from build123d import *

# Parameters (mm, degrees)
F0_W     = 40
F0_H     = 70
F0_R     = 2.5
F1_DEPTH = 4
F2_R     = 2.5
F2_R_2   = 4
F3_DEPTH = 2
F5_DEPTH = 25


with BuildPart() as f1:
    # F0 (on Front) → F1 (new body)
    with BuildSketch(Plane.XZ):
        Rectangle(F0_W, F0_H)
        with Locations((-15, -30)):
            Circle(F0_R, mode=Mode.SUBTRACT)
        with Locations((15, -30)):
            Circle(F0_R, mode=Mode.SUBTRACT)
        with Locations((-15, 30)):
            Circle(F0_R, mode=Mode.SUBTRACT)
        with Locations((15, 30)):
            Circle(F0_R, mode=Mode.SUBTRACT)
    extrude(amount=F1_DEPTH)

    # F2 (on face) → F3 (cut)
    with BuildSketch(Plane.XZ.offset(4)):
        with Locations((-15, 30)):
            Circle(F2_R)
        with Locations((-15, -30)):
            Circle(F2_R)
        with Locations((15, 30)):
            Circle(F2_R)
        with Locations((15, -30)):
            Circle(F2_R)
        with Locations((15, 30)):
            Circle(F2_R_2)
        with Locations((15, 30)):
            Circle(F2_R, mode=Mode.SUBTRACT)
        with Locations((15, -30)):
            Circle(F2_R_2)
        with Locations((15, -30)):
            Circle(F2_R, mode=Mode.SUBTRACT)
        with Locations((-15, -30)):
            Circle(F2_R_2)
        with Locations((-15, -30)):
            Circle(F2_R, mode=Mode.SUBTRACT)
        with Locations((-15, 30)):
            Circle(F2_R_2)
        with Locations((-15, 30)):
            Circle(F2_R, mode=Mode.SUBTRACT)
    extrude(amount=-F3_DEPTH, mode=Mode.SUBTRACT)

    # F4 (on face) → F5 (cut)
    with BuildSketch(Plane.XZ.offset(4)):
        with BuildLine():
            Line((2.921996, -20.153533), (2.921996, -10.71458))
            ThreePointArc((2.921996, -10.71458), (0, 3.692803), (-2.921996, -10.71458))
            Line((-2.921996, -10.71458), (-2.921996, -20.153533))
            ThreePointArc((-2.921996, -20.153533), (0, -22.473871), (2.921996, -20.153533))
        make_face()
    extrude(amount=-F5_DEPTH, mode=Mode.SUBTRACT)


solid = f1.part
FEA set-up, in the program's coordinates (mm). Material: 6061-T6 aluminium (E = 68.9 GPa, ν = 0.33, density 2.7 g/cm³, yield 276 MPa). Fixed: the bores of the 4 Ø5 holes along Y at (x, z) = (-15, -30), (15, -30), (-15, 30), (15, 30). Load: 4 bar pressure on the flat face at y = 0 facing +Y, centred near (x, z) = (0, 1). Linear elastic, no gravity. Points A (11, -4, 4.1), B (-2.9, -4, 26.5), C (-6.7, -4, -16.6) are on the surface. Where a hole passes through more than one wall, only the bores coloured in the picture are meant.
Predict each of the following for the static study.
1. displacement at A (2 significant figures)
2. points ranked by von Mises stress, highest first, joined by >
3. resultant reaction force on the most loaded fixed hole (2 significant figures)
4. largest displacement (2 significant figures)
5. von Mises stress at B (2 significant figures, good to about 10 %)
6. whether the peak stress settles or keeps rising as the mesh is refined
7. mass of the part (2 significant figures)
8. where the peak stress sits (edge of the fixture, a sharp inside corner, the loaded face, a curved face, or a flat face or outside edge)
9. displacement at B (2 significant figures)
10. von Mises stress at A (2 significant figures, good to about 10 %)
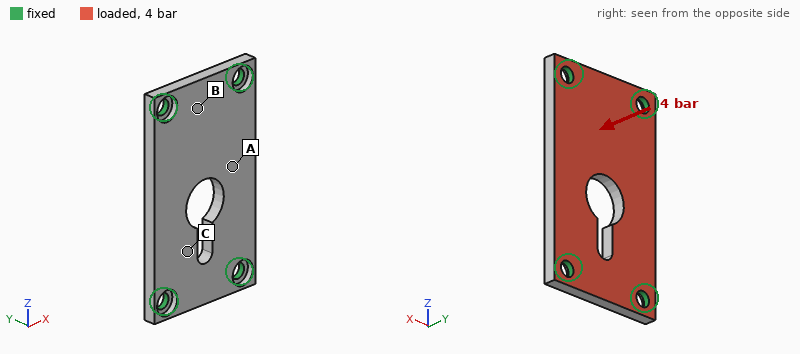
54 µm
A > B > C
360 N
60 µm
15 MPa
keeps rising
26 g
edge of the fixture
12 µm
29 MPa
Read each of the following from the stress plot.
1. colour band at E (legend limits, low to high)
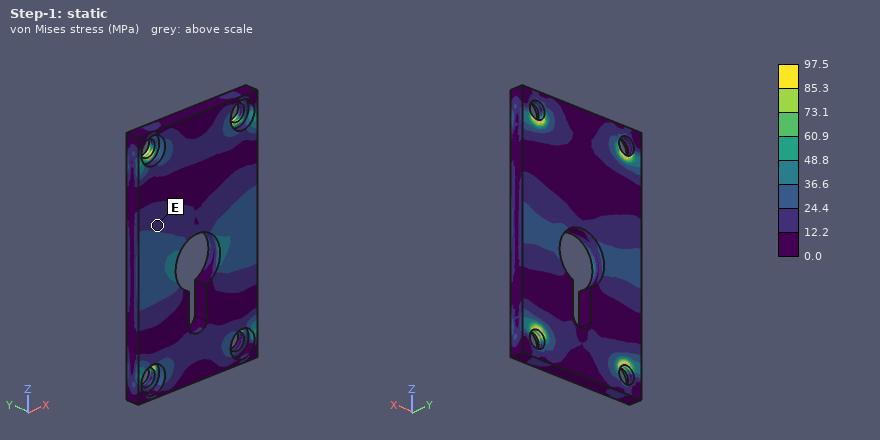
12.2 to 24.4 MPa
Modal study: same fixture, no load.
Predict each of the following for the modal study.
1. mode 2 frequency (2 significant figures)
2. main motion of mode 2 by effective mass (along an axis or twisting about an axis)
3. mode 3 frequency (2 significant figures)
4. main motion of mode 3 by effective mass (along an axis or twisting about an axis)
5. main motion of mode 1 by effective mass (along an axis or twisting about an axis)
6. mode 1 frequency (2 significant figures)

6800 Hz
twisting about Z
12 kHz
twisting about X
along Y
4700 Hz
